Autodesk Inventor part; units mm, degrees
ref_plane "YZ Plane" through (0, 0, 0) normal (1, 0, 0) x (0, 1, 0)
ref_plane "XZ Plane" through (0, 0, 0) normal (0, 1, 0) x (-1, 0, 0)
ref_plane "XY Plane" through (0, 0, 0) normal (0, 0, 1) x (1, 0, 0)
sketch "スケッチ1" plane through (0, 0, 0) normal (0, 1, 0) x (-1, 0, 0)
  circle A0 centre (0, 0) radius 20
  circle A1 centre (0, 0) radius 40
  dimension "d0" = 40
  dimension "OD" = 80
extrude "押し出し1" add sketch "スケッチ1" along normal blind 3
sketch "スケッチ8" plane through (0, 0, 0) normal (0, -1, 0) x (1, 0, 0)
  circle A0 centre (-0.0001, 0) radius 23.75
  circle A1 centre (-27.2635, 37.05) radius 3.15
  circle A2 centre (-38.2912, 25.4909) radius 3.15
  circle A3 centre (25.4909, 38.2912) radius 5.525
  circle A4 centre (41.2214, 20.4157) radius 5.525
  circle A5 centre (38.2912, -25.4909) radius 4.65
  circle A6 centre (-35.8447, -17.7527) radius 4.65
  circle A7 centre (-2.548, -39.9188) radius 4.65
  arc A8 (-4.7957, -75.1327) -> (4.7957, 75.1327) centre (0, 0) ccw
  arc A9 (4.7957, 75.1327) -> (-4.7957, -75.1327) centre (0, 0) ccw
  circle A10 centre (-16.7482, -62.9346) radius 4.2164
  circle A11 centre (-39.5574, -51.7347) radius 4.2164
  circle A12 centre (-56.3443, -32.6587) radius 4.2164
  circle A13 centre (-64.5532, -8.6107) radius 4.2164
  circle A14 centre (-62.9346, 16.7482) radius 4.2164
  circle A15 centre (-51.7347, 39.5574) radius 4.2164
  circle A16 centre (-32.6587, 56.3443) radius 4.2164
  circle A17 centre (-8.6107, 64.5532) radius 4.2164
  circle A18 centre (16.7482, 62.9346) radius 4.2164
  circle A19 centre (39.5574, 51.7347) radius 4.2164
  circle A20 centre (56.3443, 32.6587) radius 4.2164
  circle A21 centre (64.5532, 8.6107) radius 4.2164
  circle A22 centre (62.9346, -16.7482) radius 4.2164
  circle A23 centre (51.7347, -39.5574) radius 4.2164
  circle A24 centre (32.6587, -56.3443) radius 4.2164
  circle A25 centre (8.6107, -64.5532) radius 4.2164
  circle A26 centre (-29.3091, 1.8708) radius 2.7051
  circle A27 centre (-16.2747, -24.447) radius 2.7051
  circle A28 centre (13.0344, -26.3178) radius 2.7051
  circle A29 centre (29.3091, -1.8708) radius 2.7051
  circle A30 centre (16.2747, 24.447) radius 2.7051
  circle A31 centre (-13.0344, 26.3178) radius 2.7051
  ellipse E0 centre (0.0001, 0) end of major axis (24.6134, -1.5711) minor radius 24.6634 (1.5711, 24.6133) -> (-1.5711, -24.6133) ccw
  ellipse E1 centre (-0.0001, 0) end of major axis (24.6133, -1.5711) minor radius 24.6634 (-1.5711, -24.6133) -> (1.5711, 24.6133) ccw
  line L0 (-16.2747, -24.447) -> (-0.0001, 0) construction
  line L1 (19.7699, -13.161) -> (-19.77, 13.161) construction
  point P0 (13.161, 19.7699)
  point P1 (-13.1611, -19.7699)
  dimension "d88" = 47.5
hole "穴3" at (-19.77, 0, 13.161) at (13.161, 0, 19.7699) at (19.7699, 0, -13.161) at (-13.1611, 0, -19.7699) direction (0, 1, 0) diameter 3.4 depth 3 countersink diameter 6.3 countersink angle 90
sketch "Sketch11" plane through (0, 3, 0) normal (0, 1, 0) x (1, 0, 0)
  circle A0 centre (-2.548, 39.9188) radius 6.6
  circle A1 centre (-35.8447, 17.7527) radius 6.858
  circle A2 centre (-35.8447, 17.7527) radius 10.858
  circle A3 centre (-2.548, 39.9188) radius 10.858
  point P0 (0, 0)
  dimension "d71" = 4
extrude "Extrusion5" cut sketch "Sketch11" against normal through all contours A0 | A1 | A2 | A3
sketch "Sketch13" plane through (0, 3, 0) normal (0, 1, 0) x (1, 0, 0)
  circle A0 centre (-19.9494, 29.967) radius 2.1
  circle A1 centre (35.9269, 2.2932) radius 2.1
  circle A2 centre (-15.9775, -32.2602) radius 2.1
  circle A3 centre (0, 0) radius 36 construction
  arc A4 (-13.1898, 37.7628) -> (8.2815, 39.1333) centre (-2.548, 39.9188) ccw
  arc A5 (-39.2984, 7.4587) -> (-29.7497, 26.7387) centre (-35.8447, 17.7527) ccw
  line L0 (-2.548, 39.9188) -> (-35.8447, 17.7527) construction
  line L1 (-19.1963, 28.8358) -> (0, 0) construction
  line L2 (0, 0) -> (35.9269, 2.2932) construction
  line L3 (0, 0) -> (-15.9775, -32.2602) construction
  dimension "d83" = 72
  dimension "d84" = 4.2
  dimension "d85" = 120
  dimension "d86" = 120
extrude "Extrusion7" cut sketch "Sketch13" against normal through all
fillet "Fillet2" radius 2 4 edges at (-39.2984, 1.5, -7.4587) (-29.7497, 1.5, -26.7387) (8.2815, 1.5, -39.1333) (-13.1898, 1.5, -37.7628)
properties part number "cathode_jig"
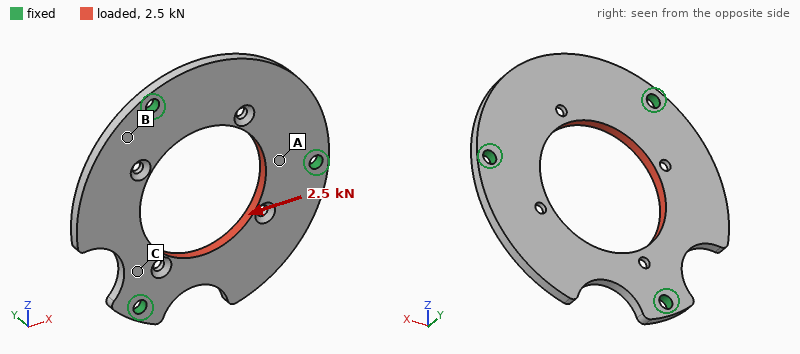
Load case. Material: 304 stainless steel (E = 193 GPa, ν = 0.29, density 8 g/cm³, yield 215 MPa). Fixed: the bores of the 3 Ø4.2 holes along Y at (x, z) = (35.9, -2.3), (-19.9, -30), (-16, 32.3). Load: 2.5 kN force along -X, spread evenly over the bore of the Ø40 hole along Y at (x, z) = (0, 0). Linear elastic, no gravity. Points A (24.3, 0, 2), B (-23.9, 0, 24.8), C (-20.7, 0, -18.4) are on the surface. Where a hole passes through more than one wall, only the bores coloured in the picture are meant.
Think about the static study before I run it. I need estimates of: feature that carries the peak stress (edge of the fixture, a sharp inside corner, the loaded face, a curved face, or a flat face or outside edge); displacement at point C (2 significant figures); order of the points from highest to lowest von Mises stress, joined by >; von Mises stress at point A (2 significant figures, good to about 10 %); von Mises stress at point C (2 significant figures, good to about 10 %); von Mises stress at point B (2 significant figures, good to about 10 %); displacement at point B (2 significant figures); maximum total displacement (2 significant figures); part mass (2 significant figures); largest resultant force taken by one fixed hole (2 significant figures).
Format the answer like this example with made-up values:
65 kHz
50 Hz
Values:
edge of the fixture
5.6 µm
C > A > B
16 MPa
26 MPa
7.9 MPa
2.3 µm
9.7 µm
80 g
950 N
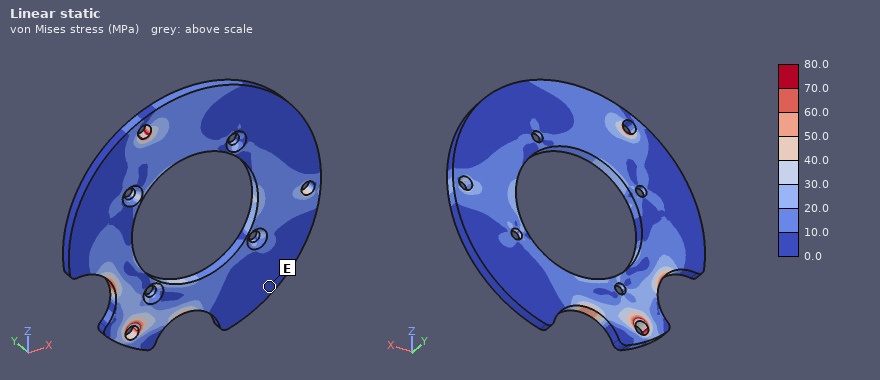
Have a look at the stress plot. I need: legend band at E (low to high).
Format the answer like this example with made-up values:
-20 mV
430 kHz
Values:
0.0 to 10.0 MPa
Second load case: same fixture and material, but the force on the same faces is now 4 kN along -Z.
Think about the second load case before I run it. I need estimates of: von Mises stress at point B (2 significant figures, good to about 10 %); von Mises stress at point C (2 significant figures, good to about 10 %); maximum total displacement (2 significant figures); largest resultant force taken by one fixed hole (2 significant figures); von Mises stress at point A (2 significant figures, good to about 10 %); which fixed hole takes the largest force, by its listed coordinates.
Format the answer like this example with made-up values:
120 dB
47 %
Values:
17 MPa
23 MPa
12 µm
1.6 kN
18 MPa
(35.9, -2.3)
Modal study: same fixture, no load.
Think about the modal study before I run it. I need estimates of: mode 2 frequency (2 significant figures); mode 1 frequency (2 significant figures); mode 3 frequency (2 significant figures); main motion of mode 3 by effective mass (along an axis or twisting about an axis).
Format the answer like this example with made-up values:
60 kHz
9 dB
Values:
2700 Hz
2600 Hz
3000 Hz
along Y
